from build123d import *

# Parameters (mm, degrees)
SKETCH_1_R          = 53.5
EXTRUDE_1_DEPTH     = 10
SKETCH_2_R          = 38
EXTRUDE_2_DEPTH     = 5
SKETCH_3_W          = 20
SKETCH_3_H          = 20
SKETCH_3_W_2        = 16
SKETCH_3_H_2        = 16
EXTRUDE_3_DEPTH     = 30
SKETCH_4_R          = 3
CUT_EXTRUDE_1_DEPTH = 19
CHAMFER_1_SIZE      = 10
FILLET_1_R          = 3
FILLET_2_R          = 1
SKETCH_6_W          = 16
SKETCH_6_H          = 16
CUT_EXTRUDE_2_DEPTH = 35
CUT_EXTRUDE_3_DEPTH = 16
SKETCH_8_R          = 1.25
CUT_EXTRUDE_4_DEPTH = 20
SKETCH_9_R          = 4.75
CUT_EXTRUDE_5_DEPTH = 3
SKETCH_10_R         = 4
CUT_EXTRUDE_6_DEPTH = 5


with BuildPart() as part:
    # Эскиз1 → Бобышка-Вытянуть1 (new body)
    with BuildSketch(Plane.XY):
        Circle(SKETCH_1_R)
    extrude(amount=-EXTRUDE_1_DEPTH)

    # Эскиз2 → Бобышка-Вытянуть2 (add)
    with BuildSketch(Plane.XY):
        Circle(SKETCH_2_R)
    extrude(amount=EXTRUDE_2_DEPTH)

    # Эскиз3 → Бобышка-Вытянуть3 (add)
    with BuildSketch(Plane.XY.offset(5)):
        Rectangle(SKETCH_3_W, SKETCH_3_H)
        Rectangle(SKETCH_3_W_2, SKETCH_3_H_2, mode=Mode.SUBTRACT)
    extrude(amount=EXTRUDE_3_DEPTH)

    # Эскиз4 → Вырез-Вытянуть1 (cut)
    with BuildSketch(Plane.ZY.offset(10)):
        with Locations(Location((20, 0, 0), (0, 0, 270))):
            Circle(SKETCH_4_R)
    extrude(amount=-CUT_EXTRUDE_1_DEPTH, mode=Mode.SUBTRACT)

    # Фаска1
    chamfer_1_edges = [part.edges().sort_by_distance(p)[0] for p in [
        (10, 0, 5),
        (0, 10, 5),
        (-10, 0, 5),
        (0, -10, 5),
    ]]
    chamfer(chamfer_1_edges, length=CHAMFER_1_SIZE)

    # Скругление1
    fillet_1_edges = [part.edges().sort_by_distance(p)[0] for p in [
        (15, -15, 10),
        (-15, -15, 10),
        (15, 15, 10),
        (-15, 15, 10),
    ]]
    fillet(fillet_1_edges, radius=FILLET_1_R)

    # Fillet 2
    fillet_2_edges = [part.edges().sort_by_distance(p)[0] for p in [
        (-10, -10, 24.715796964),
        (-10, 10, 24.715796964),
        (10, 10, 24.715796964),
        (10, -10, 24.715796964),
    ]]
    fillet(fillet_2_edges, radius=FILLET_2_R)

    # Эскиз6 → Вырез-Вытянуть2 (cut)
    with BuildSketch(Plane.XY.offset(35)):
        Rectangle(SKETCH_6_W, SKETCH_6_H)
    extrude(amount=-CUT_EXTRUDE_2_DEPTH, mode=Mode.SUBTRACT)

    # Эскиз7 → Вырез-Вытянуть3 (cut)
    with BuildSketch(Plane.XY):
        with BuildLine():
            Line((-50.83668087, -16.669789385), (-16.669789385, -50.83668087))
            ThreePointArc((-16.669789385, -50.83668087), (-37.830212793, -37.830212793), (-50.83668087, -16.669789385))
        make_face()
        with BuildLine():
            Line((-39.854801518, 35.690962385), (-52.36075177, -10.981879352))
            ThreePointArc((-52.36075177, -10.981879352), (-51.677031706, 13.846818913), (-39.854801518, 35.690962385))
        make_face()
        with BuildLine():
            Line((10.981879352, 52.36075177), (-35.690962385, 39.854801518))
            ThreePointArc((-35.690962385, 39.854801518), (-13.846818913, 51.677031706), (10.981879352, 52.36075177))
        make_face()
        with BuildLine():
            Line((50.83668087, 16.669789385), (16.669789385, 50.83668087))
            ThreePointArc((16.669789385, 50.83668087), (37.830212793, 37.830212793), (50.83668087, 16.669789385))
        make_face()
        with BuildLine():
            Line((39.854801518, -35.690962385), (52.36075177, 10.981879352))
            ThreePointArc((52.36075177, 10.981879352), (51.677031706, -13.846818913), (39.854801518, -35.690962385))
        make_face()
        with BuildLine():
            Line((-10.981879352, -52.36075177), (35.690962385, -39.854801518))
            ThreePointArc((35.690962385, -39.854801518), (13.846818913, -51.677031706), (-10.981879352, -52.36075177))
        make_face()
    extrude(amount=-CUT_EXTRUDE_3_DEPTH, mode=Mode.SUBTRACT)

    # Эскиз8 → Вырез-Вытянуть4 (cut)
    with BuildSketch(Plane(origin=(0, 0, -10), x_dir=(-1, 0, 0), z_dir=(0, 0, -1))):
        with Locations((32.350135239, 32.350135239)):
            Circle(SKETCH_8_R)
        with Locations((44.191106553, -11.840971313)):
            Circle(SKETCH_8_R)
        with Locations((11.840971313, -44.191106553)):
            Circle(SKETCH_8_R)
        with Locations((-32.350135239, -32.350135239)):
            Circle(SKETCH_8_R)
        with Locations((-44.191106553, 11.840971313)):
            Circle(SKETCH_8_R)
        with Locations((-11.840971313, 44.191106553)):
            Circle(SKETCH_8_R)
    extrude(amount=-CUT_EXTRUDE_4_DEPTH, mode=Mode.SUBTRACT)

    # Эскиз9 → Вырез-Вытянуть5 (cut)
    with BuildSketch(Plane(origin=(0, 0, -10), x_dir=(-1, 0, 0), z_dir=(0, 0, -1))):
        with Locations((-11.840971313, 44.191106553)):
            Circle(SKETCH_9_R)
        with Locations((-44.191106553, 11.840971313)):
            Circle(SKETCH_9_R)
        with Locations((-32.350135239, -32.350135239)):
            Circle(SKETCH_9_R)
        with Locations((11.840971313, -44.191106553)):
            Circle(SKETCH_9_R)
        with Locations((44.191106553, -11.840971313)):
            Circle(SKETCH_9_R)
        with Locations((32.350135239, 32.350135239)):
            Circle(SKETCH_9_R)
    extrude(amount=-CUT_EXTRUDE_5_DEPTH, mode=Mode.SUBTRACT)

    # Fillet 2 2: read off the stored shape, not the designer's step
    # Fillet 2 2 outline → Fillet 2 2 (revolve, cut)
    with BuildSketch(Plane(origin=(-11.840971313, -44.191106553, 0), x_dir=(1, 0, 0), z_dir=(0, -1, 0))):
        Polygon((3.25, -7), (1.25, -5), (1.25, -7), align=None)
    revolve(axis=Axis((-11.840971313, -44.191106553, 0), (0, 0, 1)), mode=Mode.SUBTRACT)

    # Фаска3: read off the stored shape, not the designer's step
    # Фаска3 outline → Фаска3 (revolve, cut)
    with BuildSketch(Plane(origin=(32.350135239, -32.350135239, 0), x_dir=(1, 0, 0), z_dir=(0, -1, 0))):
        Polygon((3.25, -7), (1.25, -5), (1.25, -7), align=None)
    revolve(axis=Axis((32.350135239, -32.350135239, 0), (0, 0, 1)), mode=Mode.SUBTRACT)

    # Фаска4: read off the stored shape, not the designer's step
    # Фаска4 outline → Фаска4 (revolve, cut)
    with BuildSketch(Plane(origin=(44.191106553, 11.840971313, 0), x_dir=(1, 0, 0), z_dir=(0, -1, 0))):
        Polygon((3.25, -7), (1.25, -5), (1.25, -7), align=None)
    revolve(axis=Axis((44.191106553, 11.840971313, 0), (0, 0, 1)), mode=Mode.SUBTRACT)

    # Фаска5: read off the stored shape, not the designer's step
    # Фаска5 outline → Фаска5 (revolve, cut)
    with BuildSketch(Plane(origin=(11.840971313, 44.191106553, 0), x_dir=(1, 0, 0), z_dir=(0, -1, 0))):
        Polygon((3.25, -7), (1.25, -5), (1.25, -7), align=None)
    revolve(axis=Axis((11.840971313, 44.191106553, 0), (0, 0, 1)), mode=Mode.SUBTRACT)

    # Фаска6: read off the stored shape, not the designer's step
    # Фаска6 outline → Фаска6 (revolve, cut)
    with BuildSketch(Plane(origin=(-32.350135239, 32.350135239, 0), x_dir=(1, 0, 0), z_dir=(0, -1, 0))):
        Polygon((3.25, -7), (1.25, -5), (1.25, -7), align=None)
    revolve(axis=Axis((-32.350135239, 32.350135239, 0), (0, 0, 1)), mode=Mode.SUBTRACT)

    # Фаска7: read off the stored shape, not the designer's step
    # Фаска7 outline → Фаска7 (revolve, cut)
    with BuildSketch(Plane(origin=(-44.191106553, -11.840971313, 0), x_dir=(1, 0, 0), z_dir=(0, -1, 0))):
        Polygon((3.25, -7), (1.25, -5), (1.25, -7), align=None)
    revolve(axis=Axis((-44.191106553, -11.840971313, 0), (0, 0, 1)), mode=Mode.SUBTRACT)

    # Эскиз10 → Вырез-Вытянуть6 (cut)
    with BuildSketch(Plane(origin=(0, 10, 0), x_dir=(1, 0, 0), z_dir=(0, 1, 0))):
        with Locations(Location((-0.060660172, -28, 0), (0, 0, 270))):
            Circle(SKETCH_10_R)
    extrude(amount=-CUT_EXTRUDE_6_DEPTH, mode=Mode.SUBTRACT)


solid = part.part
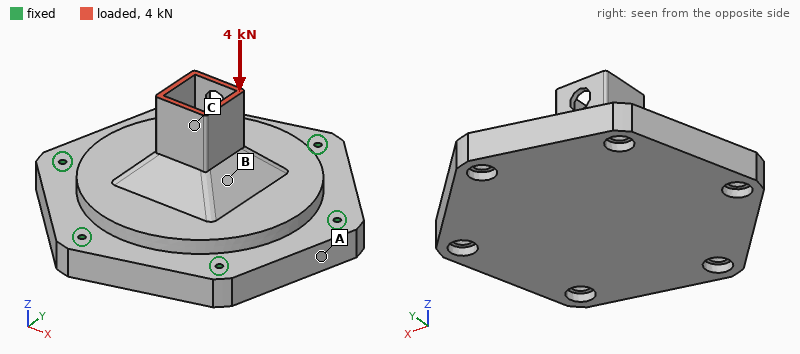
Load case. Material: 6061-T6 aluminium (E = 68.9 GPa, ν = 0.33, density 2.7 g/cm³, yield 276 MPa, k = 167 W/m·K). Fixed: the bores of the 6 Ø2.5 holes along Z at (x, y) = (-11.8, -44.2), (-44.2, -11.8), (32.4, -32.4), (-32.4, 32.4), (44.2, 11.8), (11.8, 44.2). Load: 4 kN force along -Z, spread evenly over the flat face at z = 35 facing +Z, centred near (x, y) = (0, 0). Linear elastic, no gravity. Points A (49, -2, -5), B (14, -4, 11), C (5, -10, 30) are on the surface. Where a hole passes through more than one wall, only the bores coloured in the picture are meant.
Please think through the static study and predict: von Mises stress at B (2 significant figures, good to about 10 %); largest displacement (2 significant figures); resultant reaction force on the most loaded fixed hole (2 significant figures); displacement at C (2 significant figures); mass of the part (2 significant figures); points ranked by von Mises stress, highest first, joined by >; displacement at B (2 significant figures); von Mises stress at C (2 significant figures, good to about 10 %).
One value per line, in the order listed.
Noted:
11 MPa
33 µm
670 N
21 µm
290 g
C > B > A
13 µm
28 MPa
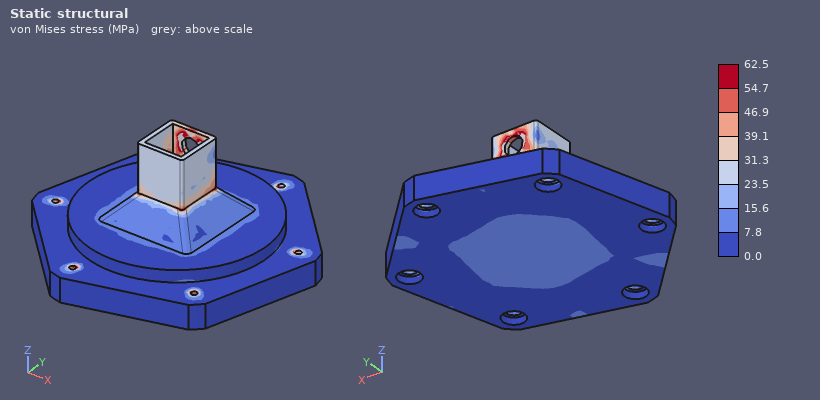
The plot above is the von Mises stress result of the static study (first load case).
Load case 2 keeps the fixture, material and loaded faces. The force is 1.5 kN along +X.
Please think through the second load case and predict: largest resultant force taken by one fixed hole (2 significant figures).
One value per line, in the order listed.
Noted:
500 N
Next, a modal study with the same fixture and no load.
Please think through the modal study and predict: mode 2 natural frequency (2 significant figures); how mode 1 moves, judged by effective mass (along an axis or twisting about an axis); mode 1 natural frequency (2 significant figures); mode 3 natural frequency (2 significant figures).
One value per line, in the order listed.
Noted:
12 kHz
along Z
7200 Hz
12 kHz
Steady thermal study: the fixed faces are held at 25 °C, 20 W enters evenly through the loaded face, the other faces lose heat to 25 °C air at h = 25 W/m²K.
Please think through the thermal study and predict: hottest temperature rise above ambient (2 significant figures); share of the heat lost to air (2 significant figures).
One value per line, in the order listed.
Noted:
27 K
9.5 %
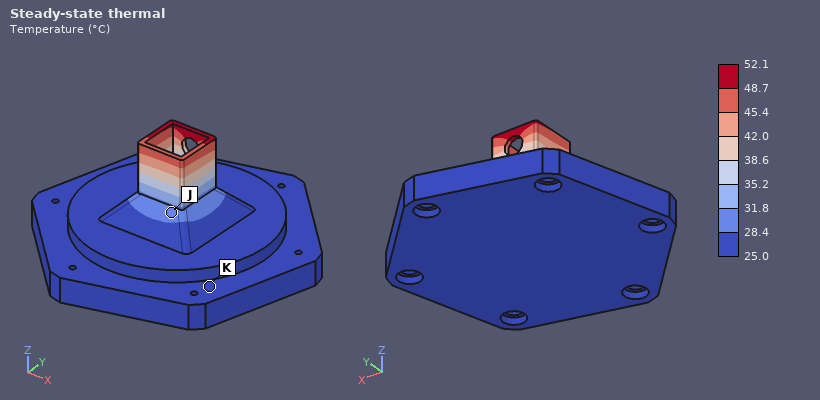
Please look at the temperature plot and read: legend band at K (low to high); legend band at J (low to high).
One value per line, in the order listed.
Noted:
25.0 to 28.4 °C
28.4 to 31.8 °C
